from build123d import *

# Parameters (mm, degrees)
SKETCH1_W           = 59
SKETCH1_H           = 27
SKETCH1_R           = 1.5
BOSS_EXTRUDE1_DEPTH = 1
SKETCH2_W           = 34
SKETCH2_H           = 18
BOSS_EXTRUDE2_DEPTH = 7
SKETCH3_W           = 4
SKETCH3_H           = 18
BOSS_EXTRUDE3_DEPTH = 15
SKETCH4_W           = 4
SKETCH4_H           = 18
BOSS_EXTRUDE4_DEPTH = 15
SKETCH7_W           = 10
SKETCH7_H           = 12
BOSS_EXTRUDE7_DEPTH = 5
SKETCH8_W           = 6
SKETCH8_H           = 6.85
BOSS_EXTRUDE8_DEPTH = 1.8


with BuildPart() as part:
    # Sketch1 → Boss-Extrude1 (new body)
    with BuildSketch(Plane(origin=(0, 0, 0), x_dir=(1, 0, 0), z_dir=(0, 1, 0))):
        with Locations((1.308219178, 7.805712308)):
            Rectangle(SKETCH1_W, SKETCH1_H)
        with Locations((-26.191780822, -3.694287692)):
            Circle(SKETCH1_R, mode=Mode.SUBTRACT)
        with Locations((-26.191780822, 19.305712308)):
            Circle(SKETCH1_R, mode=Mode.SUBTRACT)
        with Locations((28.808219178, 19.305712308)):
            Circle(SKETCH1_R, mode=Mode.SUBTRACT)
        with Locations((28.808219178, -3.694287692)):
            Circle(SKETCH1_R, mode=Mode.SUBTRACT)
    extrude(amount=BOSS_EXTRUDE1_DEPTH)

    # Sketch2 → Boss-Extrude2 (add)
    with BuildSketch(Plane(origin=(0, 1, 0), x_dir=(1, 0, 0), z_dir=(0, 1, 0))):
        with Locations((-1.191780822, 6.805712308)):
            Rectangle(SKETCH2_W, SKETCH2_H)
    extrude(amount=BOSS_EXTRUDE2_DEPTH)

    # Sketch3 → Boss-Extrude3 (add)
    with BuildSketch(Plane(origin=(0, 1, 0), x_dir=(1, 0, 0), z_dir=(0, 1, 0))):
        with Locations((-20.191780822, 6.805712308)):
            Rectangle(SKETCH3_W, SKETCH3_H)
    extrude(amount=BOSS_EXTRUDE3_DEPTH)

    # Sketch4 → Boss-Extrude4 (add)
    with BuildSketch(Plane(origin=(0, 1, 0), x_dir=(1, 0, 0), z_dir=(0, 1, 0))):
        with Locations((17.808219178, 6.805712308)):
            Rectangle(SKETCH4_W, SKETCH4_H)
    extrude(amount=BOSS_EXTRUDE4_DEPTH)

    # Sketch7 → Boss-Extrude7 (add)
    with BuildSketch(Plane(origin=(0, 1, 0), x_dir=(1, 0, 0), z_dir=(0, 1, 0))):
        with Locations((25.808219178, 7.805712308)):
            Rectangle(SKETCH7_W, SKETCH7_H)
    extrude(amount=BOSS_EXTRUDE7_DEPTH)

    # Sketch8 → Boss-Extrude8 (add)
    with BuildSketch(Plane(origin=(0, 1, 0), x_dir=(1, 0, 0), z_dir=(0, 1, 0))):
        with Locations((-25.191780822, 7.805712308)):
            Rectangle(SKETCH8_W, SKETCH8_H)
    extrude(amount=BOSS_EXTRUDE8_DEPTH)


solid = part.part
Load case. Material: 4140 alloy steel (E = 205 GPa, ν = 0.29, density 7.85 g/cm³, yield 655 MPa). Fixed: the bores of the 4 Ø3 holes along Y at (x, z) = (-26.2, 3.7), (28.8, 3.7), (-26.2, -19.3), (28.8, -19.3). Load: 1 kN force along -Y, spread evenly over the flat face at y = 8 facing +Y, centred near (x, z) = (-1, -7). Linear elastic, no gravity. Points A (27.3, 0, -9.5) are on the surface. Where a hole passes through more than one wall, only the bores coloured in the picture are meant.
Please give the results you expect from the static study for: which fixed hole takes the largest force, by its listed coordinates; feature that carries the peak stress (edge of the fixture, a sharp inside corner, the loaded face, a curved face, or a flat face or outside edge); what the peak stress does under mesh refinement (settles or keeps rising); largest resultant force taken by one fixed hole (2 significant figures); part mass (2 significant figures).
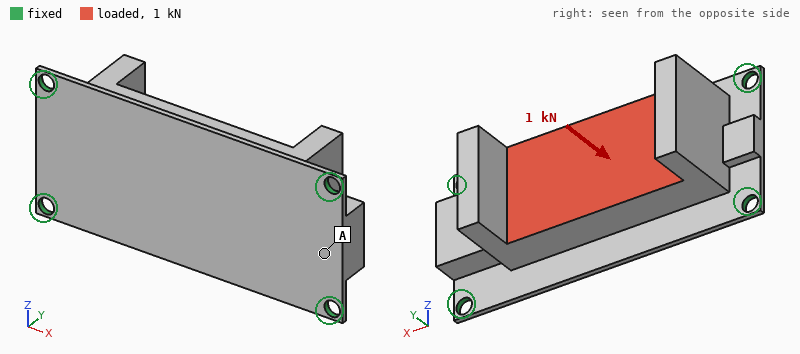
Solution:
(-26.2, 3.7)
edge of the fixture
keeps rising
470 N
68 g
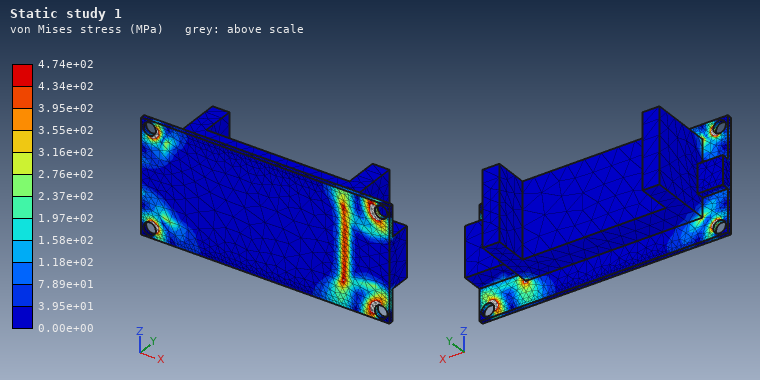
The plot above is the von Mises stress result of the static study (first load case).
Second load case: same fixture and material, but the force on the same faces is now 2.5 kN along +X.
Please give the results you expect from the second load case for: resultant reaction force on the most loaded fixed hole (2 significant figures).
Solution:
770 N
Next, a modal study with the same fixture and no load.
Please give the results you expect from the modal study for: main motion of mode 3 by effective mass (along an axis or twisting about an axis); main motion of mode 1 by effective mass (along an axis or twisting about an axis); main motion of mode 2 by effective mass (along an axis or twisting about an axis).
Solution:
along Y
along Y
along Z
